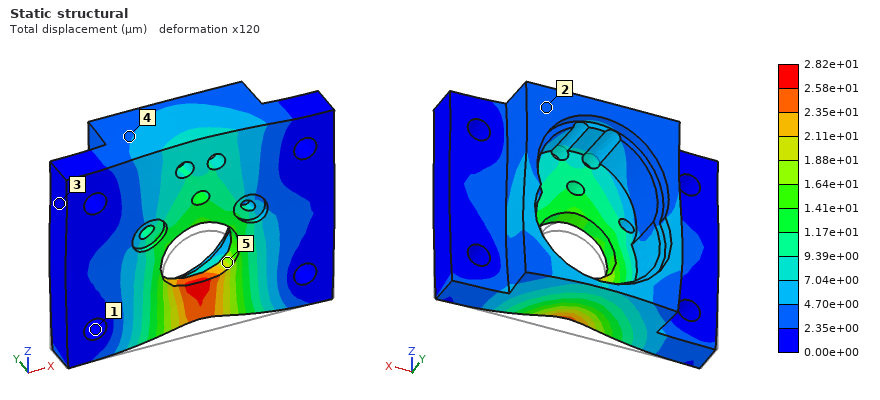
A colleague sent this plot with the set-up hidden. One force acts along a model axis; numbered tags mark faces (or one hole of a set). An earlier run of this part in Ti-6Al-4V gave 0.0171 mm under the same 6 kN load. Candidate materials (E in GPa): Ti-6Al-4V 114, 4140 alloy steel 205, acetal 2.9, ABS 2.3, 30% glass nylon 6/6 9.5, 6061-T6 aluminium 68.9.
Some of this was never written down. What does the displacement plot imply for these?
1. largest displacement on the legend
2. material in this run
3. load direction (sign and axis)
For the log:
2.82e+01 µm
6061-T6 aluminium
+Z
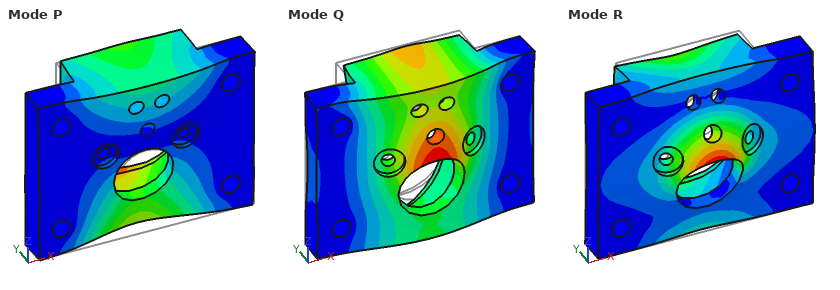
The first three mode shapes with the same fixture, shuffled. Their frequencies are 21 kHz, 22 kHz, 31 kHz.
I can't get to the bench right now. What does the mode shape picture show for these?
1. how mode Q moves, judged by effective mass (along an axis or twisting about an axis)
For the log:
along Y
